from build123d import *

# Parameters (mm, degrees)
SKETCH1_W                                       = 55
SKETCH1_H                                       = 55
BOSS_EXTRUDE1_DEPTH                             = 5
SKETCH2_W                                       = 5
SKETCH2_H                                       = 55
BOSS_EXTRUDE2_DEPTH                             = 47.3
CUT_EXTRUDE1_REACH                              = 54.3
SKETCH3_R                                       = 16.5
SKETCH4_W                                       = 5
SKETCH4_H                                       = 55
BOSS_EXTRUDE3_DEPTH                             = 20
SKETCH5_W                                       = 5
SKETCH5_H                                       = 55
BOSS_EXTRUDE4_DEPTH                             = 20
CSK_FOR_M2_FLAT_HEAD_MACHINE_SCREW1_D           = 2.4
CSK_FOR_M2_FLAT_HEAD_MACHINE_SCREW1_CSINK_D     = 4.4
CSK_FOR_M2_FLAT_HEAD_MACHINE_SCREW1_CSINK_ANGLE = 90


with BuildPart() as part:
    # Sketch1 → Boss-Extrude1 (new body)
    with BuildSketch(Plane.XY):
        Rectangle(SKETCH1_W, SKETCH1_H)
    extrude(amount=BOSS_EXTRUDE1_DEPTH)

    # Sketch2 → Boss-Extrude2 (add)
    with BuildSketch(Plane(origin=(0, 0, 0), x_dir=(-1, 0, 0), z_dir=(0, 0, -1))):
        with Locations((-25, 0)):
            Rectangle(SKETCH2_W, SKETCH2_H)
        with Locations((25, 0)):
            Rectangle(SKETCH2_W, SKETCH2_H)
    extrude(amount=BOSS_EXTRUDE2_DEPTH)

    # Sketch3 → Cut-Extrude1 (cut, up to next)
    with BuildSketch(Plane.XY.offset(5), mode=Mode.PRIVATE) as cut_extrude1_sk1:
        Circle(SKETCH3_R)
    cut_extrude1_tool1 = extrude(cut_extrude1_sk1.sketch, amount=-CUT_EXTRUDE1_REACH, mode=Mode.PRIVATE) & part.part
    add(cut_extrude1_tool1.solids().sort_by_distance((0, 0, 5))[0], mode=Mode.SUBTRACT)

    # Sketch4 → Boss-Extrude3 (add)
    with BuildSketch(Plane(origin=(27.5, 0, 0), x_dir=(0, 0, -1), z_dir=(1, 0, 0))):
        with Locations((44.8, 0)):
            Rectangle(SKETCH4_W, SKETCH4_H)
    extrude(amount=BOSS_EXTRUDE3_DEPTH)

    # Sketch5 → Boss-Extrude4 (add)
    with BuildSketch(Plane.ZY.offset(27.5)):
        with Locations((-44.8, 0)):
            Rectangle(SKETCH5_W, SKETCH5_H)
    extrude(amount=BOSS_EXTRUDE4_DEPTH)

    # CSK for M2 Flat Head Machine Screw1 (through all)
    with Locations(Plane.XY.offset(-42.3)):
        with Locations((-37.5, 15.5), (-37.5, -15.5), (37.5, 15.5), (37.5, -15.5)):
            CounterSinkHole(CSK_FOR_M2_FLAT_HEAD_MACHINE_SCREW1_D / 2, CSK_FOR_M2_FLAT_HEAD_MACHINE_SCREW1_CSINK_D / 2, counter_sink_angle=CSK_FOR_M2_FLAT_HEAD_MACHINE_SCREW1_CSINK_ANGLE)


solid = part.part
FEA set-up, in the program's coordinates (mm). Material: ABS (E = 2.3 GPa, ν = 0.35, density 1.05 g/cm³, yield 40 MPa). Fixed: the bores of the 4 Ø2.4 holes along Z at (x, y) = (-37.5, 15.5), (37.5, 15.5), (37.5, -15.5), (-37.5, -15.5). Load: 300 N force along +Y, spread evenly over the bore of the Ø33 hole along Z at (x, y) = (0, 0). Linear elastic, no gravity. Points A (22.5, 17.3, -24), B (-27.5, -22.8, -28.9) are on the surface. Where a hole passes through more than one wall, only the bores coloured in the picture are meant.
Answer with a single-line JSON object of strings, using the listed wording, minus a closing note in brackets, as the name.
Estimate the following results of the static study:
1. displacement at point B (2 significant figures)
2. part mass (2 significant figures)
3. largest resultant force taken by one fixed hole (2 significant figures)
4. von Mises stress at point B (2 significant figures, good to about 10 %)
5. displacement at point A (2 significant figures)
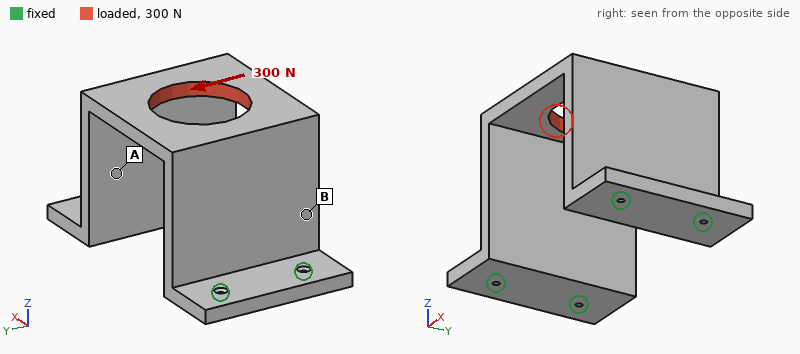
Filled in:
{"displacement at point B": "0.41 mm", "part mass": "50 g", "largest resultant force taken by one fixed hole": "240 N", "von Mises stress at point B": "4.8 MPa", "displacement at point A": "0.38 mm"}
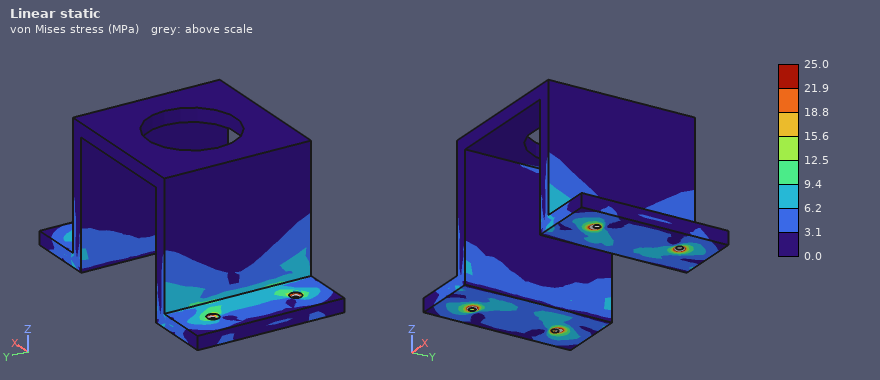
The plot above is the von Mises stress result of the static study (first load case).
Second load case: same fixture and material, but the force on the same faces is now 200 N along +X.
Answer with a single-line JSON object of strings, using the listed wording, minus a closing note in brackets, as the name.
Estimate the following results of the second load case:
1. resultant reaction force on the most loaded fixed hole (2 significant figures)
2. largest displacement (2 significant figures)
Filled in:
{"resultant reaction force on the most loaded fixed hole": "71 N", "largest displacement": "1.4 mm"}
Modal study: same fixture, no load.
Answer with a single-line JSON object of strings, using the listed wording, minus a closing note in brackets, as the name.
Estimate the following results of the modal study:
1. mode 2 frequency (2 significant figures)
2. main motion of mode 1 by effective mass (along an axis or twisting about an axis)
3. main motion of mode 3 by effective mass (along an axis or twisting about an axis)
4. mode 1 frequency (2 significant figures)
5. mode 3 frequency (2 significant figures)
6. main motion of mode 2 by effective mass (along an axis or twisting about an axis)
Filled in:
{"mode 2 frequency": "680 Hz", "main motion of mode 1 by effective mass": "along X", "main motion of mode 3 by effective mass": "twisting about Z", "mode 1 frequency": "420 Hz", "mode 3 frequency": "720 Hz", "main motion of mode 2 by effective mass": "along Y"}
